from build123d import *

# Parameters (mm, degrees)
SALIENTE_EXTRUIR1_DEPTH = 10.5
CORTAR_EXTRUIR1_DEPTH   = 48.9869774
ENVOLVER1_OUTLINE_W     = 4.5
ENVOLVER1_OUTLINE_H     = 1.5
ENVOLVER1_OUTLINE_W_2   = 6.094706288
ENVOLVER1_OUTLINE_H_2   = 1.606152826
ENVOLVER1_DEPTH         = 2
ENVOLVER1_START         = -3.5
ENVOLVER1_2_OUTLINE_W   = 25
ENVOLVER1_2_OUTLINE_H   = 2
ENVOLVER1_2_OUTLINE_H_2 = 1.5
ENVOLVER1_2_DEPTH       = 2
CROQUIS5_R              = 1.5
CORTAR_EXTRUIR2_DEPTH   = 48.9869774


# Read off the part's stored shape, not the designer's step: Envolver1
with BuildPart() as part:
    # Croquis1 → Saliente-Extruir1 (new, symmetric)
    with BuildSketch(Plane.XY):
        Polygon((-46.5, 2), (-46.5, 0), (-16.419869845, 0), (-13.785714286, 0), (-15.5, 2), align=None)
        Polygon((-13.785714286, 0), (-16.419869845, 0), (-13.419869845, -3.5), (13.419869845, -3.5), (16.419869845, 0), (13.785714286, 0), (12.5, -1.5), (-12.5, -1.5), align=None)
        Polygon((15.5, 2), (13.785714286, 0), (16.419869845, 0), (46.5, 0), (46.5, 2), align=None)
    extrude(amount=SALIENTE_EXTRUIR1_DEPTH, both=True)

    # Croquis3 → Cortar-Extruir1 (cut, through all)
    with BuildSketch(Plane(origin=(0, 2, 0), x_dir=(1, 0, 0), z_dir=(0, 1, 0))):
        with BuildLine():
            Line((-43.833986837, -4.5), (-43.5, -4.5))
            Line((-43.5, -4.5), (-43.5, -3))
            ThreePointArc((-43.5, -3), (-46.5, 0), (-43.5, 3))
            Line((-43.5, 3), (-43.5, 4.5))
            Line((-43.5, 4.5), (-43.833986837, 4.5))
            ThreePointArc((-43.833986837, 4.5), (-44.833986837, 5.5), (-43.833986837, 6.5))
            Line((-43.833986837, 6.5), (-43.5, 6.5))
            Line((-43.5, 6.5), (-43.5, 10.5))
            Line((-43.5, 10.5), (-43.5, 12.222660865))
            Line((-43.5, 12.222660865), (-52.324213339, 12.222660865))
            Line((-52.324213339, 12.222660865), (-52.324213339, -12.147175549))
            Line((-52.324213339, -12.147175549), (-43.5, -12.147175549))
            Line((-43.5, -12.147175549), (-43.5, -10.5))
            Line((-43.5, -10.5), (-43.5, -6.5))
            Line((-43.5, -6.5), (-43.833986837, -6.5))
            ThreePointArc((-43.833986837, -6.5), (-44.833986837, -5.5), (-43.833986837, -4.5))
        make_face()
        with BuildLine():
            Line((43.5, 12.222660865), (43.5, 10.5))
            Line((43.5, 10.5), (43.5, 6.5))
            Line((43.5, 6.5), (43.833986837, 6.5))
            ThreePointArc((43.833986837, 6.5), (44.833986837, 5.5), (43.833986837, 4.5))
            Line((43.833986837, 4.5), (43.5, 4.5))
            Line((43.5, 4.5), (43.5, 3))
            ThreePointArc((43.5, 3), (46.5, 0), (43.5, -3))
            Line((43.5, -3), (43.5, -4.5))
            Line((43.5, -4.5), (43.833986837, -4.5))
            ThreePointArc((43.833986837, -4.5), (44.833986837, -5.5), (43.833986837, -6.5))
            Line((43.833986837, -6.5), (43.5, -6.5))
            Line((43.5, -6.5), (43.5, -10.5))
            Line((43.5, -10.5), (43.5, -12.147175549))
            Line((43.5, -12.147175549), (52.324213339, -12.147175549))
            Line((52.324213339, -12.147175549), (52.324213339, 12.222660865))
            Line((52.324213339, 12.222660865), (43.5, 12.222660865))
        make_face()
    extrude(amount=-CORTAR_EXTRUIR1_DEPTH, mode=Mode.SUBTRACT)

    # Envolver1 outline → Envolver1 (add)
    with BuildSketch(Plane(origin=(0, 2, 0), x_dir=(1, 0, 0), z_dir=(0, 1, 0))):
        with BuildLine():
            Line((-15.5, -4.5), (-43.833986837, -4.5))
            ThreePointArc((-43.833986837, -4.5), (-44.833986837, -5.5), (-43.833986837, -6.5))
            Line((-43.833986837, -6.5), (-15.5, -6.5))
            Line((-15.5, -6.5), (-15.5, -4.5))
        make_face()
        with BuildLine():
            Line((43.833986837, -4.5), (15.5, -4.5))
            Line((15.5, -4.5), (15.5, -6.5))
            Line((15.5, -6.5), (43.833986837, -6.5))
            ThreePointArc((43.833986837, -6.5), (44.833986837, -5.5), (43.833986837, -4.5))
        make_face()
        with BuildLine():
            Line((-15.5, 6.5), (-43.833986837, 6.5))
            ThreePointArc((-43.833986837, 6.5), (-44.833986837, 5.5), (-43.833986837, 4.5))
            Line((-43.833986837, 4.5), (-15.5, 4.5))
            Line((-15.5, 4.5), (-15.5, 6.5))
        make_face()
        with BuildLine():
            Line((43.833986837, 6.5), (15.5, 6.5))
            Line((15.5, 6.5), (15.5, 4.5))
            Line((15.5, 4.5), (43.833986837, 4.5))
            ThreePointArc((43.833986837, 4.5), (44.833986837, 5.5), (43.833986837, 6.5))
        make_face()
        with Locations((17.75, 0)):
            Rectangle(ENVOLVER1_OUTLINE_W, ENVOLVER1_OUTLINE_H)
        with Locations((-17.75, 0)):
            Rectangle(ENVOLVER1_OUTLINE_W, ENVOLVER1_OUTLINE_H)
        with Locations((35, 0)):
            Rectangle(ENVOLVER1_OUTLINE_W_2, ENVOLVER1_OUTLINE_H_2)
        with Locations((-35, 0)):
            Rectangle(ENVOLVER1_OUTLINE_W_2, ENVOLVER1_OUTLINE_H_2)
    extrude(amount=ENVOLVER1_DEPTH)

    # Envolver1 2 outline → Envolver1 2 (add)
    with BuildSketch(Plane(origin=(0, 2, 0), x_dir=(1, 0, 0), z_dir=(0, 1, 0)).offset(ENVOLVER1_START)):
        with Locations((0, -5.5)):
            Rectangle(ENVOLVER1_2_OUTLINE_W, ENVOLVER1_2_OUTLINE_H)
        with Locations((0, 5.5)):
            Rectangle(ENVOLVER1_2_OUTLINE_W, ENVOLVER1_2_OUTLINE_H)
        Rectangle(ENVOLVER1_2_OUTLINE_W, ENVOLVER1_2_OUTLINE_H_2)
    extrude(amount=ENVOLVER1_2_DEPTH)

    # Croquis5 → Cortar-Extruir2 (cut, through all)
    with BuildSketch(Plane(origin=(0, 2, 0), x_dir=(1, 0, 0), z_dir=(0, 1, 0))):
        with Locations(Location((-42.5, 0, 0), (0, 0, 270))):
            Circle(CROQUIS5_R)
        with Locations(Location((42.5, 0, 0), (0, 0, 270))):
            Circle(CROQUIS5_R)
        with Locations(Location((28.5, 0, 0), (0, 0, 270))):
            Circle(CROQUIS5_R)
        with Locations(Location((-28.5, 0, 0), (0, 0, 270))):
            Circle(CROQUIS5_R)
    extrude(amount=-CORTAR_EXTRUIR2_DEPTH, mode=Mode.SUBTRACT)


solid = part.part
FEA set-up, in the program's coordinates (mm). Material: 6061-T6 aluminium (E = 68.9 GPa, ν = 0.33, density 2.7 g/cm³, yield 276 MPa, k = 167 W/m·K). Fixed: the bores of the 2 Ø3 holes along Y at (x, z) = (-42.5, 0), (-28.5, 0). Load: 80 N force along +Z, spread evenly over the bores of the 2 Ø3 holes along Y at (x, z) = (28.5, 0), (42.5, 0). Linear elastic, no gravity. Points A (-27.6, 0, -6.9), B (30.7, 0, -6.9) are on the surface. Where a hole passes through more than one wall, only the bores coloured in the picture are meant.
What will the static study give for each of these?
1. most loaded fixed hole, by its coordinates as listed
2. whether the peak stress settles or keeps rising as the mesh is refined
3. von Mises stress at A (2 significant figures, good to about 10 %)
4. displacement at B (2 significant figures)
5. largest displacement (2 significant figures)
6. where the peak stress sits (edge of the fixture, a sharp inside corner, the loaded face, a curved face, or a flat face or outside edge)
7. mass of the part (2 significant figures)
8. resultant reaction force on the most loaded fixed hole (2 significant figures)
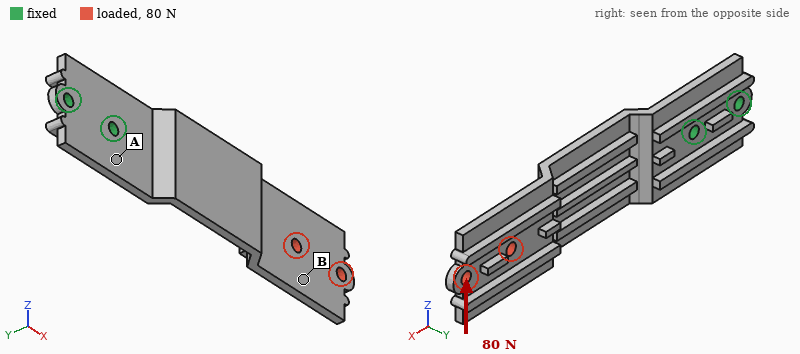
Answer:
(-28.5, 0)
keeps rising
30 MPa
0.22 mm
0.31 mm
a sharp inside corner
12 g
380 N
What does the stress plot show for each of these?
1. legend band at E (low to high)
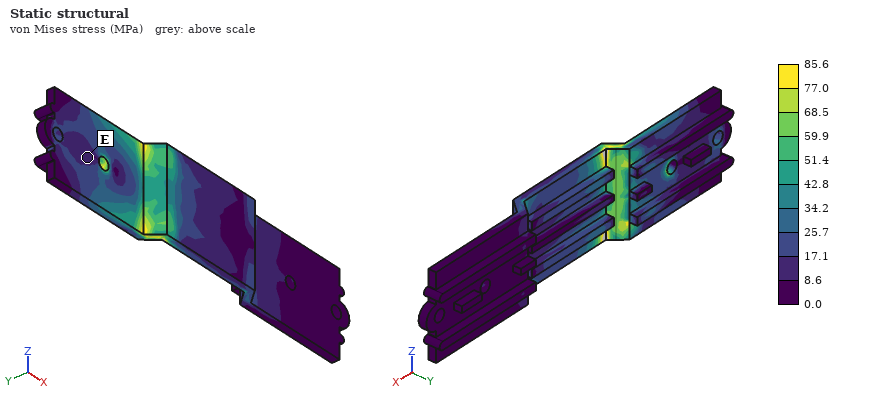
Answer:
8.6 to 17.1 MPa
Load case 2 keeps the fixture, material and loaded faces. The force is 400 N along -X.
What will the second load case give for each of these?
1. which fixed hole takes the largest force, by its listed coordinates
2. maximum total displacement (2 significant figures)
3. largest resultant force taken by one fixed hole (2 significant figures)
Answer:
(-28.5, 0)
0.80 mm
310 N
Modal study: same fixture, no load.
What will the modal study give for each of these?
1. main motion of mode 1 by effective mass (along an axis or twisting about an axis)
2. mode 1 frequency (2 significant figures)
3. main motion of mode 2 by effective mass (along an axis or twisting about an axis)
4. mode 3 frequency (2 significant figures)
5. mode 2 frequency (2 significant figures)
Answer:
along Y
390 Hz
along Z
2400 Hz
1400 Hz
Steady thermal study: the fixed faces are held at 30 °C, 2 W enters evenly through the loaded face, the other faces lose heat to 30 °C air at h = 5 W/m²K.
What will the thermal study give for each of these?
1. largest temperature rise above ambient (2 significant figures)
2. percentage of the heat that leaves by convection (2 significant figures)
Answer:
17 K
9.6 %
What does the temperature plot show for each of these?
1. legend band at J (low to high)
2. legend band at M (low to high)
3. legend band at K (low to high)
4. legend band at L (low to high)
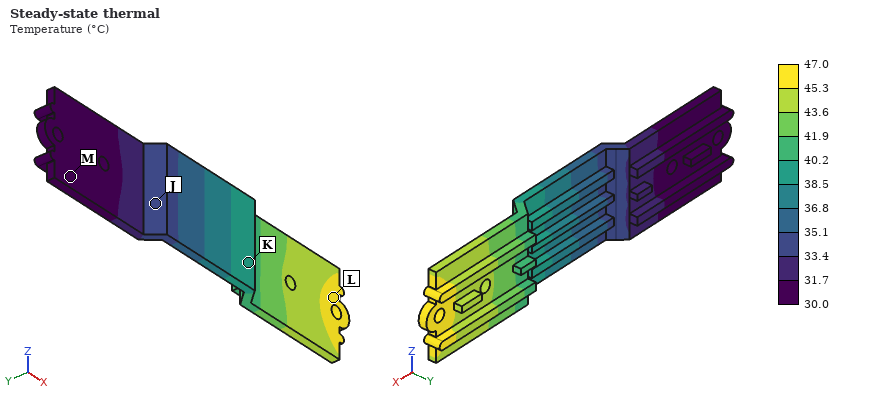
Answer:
33.4 to 35.1 °C
30.0 to 31.7 °C
38.5 to 40.2 °C
45.3 to 47.0 °C
